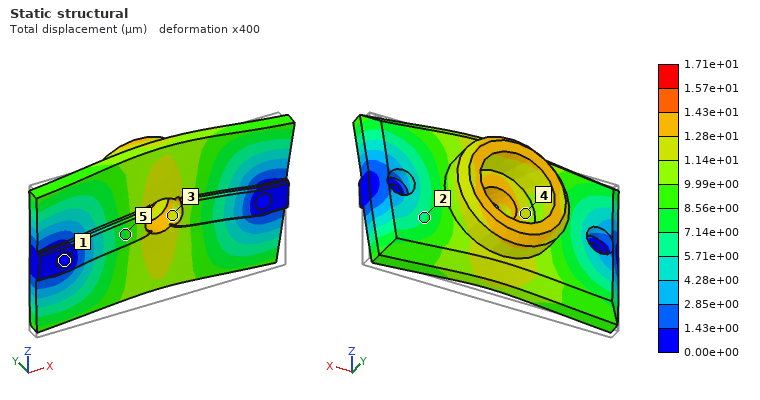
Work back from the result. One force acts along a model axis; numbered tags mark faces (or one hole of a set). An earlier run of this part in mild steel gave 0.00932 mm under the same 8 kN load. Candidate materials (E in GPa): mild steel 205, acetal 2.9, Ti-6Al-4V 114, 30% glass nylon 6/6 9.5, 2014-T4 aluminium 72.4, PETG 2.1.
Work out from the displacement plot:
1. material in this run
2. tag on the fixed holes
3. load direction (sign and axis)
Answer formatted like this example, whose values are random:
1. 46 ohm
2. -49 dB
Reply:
1. Ti-6Al-4V
2. 1
3. +Z
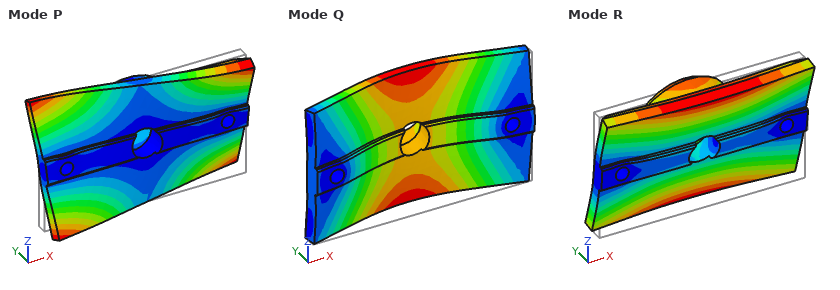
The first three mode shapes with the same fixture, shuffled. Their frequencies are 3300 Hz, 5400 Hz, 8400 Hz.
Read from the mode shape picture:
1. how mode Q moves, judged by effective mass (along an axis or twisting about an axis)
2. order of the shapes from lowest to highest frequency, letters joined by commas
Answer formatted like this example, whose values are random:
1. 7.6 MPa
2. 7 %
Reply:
1. along Y
2. R, Q, P
